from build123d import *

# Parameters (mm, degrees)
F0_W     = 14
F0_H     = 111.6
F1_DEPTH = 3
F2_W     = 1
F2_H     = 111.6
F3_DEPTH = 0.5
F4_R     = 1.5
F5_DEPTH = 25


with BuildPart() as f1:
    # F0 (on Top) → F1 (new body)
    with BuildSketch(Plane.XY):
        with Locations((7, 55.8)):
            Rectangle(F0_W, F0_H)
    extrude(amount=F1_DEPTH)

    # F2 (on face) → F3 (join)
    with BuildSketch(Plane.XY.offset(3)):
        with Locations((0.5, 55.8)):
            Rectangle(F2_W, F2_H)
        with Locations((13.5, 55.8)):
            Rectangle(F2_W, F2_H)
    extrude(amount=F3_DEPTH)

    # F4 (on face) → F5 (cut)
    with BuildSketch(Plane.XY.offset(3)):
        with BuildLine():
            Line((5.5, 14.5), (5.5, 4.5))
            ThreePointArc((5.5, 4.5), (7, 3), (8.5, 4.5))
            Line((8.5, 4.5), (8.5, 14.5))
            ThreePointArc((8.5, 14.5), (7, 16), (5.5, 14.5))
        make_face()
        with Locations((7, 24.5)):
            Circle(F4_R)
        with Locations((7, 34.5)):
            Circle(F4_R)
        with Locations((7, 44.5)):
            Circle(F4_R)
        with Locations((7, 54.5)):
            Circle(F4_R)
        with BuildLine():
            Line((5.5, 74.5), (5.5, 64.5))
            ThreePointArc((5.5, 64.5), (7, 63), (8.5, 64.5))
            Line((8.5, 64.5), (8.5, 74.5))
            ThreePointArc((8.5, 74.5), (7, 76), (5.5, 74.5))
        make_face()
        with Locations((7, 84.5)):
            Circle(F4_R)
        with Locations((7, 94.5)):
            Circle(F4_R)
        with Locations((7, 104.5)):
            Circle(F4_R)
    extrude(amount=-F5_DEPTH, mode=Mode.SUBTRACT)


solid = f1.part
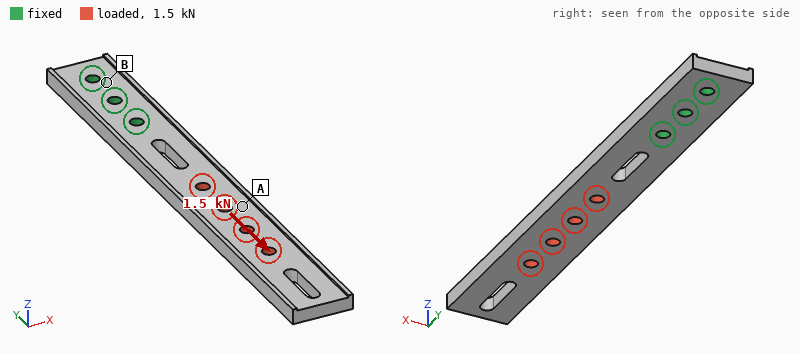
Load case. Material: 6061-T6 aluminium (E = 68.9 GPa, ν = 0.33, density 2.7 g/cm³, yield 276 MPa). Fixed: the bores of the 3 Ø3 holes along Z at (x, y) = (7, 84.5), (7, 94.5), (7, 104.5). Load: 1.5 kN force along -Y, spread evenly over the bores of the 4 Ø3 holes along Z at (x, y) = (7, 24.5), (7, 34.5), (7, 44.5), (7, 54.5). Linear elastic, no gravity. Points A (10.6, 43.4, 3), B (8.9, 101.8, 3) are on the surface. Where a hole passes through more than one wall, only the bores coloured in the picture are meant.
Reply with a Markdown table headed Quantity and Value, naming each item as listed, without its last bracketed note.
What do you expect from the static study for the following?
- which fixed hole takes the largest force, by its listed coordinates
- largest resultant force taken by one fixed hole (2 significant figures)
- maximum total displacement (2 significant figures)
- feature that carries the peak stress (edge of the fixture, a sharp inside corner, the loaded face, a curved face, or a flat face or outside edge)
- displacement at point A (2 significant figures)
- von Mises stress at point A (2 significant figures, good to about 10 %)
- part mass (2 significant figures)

| Quantity | Value |
|---|---|
| which fixed hole takes the largest force, by its listed coordinates | (7, 84.5) |
| largest resultant force taken by one fixed hole | 1.2 kN |
| maximum total displacement | 90 µm |
| feature that carries the peak stress | the loaded face |
| displacement at point A | 33 µm |
| von Mises stress at point A | 22 MPa |
| part mass | 12 g |
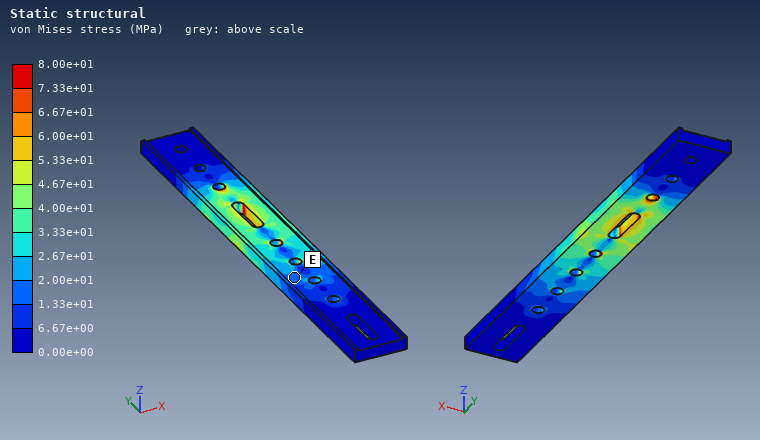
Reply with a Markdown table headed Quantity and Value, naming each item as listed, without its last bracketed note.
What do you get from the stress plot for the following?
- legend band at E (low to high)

| Quantity | Value |
|---|---|
| legend band at E | 1.33e+01 to 2.00e+01 MPa |
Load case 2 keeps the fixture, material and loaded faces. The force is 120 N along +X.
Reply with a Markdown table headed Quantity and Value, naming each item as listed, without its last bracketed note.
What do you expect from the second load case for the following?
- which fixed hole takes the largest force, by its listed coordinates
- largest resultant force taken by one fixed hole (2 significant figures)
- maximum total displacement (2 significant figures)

| Quantity | Value |
|---|---|
| which fixed hole takes the largest force, by its listed coordinates | (7, 84.5) |
| largest resultant force taken by one fixed hole | 420 N |
| maximum total displacement | 0.24 mm |
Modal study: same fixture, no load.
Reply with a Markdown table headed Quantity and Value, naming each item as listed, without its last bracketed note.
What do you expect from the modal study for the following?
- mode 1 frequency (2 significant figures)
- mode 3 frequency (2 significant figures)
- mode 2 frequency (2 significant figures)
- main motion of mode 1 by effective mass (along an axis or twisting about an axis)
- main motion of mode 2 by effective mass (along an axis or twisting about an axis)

| Quantity | Value |
|---|---|
| mode 1 frequency | 360 Hz |
| mode 3 frequency | 2200 Hz |
| mode 2 frequency | 1500 Hz |
| main motion of mode 1 by effective mass | along Z |
| main motion of mode 2 by effective mass | along X |
